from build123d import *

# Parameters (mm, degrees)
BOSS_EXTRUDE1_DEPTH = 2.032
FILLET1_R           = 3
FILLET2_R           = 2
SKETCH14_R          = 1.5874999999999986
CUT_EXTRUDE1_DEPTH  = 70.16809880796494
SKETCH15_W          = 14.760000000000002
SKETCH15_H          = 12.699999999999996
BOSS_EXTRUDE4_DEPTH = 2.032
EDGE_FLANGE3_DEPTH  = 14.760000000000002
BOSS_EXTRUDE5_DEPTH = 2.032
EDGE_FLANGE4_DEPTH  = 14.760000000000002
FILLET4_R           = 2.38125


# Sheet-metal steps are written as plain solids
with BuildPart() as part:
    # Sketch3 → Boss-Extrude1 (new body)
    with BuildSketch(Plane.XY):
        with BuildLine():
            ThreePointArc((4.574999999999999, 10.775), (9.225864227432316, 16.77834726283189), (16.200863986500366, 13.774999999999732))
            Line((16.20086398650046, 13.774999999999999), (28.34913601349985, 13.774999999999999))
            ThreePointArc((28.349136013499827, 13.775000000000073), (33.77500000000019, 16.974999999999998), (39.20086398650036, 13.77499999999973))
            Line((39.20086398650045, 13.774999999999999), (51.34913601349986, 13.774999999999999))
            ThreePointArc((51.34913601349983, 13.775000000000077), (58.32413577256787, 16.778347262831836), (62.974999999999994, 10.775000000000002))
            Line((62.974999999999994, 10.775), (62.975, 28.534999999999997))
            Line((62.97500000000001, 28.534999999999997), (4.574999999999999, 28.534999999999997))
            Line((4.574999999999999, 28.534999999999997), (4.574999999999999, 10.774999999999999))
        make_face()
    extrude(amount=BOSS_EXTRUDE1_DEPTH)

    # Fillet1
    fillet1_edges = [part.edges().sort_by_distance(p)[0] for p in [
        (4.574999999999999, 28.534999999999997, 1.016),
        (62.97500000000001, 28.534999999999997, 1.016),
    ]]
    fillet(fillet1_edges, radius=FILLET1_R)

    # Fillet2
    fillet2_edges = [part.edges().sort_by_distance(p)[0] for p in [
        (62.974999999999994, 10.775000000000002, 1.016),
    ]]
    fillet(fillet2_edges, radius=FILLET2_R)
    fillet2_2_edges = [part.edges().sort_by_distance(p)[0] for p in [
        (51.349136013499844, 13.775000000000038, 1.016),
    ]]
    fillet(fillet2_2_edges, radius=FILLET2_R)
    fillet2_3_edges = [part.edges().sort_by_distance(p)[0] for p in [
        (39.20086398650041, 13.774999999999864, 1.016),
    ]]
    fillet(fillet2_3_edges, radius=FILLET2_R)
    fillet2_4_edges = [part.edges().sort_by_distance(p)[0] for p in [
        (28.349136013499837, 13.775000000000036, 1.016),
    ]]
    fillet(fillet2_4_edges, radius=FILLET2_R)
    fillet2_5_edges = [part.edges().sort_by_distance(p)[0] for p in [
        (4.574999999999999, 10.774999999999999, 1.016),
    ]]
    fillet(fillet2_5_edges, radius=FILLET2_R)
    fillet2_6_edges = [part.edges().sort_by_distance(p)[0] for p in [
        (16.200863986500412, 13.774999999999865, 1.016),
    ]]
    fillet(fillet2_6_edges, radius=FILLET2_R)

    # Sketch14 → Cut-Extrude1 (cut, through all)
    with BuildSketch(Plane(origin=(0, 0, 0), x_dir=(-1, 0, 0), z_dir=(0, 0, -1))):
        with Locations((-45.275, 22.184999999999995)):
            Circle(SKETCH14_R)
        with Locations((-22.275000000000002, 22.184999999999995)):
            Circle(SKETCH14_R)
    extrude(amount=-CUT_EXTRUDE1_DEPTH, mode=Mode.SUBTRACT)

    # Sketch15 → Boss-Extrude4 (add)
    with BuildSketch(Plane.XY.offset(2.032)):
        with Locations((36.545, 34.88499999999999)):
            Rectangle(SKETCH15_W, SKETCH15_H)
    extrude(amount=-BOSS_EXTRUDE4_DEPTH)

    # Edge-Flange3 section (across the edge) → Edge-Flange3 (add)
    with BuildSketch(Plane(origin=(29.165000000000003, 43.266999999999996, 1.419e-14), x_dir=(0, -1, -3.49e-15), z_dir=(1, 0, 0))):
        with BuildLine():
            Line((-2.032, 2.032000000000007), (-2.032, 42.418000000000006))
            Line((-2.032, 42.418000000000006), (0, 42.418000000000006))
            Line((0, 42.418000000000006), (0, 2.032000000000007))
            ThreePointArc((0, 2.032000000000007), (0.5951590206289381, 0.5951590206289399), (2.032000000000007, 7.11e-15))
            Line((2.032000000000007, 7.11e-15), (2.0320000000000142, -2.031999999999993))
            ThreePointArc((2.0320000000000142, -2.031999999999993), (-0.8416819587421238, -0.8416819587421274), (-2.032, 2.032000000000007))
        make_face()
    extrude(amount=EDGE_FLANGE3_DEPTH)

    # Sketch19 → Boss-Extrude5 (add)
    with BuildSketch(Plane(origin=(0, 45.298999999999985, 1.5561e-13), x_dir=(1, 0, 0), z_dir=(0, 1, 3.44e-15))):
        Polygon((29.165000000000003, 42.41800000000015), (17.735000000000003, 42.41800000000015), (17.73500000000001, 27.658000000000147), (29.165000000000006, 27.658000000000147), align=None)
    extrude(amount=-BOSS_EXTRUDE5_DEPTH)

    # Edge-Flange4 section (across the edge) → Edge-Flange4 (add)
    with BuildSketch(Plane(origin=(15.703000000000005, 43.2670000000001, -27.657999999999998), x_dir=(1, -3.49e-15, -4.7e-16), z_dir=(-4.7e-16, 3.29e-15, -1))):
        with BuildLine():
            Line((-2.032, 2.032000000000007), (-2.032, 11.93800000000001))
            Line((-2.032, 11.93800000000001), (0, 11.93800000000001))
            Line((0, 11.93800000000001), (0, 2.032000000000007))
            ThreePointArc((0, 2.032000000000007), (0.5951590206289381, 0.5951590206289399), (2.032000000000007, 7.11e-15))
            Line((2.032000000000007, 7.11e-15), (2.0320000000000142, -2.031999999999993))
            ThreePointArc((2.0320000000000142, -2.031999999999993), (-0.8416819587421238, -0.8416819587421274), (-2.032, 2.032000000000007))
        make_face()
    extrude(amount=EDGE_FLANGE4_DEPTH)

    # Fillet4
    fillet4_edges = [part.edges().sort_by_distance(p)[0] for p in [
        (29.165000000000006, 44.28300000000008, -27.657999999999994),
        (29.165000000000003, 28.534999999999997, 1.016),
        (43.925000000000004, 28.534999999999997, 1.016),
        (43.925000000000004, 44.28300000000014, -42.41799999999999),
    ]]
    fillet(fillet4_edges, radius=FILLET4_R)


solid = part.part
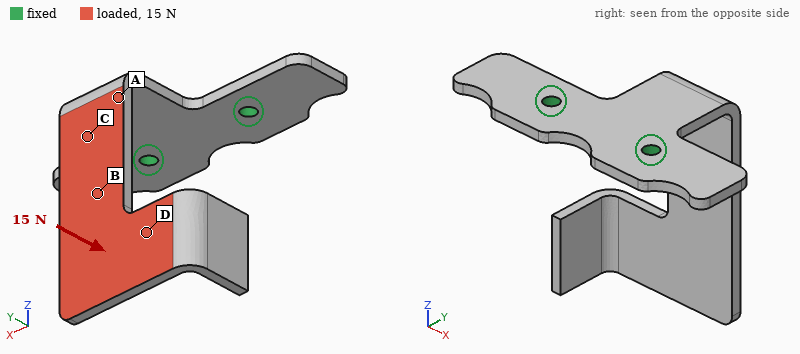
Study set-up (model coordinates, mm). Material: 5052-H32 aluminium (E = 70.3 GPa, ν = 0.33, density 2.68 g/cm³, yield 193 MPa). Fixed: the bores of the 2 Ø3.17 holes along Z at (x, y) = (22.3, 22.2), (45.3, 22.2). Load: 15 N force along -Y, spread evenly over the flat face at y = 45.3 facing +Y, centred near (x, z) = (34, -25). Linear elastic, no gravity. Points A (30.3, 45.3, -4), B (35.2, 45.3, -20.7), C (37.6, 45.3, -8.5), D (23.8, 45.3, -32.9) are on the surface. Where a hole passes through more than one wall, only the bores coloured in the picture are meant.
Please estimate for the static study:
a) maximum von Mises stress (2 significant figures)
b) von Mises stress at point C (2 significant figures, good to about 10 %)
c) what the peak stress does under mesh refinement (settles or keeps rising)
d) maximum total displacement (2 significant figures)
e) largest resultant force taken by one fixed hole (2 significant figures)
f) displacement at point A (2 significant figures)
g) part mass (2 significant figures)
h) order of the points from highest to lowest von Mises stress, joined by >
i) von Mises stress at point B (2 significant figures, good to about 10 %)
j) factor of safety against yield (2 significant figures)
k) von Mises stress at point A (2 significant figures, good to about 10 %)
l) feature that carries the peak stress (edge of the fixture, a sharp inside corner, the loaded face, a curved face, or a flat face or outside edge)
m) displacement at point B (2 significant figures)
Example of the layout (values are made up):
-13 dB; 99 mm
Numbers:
58 MPa; 23 MPa; settles; 0.74 mm; 8.4 N; 0.14 mm; 11 g; A > C > B > D; 12 MPa; 3.3; 33 MPa; a curved face; 0.34 mm
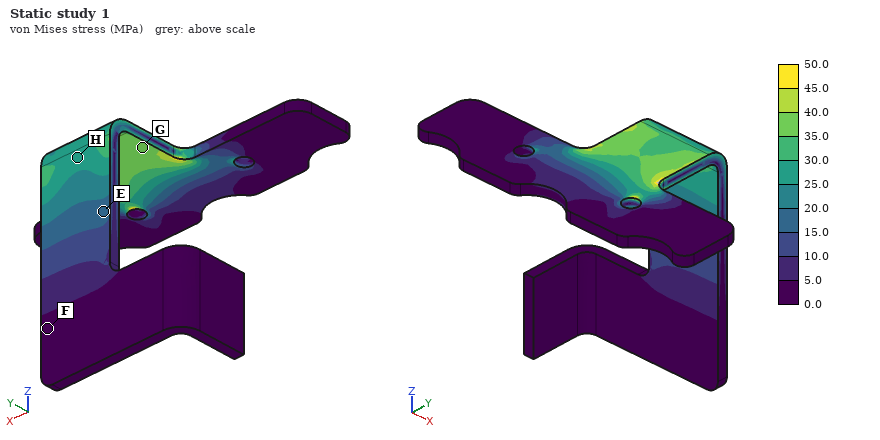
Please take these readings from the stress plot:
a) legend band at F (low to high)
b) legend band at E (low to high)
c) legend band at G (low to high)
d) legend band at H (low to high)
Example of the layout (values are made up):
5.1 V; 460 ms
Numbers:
0.0 to 5.0 MPa; 15.0 to 20.0 MPa; 35.0 to 40.0 MPa; 25.0 to 30.0 MPa
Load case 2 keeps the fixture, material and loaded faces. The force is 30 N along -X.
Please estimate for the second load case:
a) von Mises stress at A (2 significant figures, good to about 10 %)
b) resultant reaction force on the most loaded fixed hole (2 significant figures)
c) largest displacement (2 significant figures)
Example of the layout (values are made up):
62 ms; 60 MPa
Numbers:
12 MPa; 54 N; 0.57 mm
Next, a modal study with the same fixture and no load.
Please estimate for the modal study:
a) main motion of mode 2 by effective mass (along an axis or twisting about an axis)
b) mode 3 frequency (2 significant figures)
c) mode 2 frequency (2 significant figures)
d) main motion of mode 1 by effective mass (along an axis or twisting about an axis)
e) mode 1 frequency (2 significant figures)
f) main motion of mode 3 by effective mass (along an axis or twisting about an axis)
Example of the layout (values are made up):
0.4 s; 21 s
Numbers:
along X; 1200 Hz; 540 Hz; along Y; 330 Hz; along Z
